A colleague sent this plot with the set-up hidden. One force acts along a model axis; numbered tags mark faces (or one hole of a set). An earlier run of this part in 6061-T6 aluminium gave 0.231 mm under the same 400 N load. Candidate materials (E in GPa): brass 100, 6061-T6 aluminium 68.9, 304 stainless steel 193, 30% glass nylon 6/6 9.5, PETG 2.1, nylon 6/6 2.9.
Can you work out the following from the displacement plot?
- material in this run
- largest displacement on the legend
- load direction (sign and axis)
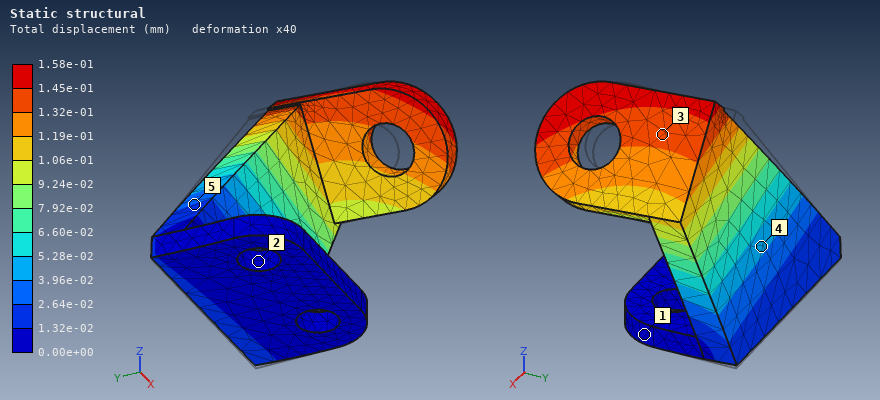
brass
1.58e-01 mm
-Y
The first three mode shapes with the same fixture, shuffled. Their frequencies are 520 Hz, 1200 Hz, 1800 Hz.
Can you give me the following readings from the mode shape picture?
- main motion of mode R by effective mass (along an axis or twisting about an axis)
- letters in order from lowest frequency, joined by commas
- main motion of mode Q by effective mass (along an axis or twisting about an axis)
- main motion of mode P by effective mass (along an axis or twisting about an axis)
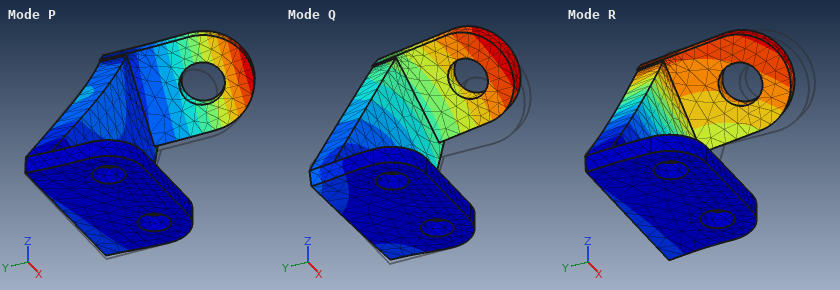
along Y
R, Q, P
along X
along Z
